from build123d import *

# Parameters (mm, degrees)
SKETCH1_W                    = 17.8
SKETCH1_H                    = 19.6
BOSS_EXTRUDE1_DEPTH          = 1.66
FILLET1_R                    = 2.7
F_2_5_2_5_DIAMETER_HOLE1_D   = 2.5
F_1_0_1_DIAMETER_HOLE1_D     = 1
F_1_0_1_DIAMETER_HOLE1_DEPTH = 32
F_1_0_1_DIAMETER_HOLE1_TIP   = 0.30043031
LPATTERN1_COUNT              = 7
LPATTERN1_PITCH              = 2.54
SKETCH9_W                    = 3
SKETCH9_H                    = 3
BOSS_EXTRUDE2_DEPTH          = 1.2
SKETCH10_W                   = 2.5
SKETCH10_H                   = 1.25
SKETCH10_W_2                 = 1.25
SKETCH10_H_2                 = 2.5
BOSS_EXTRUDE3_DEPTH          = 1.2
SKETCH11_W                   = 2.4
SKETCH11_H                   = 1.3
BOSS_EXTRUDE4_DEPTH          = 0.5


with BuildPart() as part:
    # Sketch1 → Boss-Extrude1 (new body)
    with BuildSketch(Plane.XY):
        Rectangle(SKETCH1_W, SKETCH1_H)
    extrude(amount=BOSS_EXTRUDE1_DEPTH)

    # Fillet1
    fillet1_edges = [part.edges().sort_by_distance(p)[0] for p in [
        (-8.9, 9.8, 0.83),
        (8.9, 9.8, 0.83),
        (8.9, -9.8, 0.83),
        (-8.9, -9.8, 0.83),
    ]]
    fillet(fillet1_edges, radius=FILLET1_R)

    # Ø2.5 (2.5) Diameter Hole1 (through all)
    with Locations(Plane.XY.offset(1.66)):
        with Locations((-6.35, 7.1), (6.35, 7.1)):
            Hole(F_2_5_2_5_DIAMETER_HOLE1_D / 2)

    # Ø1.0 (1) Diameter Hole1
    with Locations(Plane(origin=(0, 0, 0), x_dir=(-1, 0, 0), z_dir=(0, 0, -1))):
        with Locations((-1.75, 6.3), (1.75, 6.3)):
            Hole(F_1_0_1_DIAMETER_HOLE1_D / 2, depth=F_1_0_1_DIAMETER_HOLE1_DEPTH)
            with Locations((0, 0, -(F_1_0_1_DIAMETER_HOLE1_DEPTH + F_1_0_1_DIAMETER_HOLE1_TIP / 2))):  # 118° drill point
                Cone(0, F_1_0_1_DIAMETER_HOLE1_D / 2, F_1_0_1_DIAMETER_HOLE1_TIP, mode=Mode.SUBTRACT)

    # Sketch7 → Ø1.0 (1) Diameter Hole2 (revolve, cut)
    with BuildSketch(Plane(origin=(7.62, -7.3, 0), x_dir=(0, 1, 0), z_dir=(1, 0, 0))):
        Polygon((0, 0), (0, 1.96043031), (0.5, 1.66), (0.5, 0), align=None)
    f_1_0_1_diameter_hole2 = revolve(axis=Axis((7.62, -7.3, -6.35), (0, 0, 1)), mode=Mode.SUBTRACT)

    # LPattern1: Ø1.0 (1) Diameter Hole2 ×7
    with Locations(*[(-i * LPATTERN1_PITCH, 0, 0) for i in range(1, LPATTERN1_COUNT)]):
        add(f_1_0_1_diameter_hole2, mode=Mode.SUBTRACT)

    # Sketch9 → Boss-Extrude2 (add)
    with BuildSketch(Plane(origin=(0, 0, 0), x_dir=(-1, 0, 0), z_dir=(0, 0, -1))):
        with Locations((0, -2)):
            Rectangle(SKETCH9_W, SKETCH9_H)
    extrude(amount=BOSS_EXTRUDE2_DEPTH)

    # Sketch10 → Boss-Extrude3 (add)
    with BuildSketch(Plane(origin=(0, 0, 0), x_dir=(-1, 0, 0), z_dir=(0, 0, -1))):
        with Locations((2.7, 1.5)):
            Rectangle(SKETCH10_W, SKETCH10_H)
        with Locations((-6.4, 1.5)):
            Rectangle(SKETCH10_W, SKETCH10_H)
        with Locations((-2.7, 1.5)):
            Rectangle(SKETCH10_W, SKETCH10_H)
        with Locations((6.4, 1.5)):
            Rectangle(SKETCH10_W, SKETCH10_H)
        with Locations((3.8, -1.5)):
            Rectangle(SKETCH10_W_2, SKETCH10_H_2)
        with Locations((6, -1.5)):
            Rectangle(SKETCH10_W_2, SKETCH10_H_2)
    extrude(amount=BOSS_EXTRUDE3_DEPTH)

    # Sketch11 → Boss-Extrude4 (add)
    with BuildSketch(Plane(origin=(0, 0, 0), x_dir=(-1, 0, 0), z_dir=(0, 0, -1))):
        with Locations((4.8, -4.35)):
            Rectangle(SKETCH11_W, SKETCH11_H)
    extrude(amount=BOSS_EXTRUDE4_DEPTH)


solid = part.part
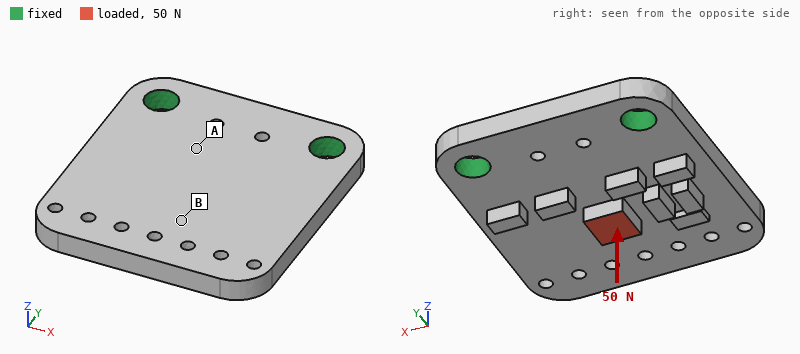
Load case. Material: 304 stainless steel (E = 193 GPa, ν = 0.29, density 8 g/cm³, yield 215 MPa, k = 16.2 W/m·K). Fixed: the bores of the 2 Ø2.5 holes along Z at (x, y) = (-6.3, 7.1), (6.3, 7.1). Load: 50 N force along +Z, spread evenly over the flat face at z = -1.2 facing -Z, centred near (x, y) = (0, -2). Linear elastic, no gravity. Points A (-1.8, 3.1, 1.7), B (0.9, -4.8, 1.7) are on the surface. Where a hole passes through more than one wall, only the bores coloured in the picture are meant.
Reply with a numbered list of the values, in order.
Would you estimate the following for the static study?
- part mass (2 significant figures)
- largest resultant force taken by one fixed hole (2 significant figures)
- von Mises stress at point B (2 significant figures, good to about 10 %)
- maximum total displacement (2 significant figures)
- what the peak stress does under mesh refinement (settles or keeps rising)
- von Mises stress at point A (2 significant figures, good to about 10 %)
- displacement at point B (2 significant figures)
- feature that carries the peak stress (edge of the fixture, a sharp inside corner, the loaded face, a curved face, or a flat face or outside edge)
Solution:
1. 4.6 g
2. 25 N
3. 12 MPa
4. 22 µm
5. keeps rising
6. 27 MPa
7. 14 µm
8. edge of the fixture
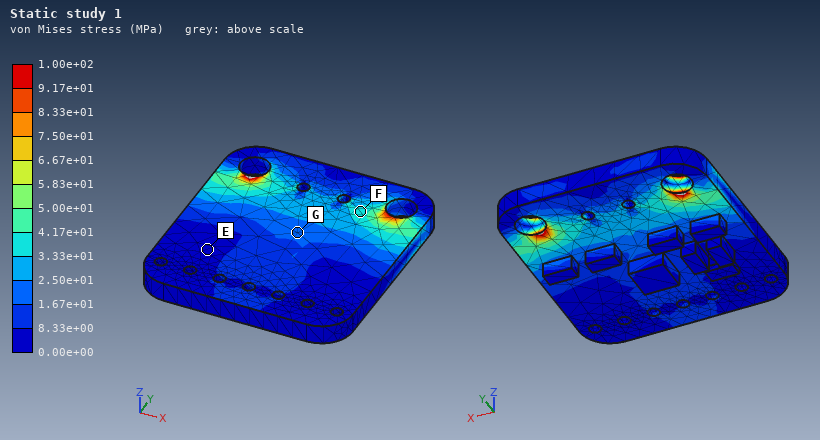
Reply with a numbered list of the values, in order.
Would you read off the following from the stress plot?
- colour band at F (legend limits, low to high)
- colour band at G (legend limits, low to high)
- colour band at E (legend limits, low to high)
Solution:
1. 3.33e+01 to 4.17e+01 MPa
2. 1.67e+01 to 2.50e+01 MPa
3. 0.00e+00 to 8.33e+00 MPa
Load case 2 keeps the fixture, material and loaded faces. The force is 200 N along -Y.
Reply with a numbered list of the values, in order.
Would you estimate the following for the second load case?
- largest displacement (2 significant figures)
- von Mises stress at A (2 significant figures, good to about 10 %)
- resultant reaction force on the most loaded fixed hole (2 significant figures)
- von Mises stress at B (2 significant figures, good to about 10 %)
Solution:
1. 32 µm
2. 36 MPa
3. 100 N
4. 23 MPa
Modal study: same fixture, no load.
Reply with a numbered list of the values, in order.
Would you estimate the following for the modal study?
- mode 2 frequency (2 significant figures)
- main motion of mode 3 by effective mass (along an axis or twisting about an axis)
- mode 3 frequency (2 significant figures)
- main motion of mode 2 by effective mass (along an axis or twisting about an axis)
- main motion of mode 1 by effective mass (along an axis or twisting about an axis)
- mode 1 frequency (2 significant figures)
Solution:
1. 12 kHz
2. along Z
3. 28 kHz
4. twisting about Y
5. along Z
6. 4900 Hz
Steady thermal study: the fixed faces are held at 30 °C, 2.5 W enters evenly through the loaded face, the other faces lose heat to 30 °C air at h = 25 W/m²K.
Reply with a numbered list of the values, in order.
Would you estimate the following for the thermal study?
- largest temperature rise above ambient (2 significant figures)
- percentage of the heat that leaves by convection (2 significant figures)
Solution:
1. 78 K
2. 23 %
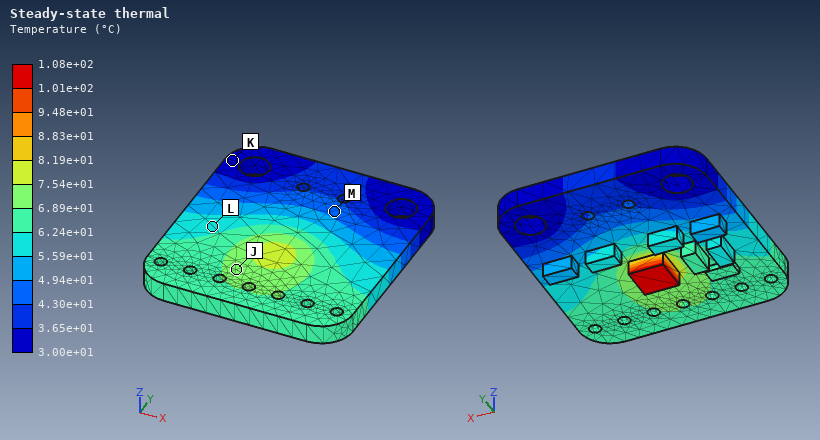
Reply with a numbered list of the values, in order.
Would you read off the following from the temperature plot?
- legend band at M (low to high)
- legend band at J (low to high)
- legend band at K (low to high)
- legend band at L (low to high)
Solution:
1. 4.30e+01 to 4.94e+01 °C
2. 6.89e+01 to 7.54e+01 °C
3. 3.00e+01 to 3.65e+01 °C
4. 5.59e+01 to 6.24e+01 °C
